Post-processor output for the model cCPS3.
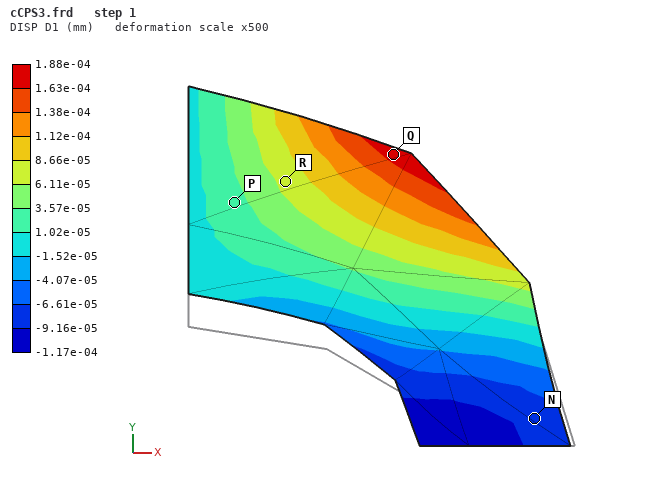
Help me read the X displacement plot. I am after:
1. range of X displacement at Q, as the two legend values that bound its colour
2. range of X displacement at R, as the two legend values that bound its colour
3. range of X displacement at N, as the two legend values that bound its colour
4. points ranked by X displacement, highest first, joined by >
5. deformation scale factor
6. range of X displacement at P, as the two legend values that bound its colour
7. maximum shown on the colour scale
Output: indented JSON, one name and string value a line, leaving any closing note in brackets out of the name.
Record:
{
  "range of X displacement at Q, as the two legend values that bound its colour": "1.63e-04 to 1.88e-04 mm",
  "range of X displacement at R, as the two legend values that bound its colour": "6.11e-05 to 8.66e-05 mm",
  "range of X displacement at N, as the two legend values that bound its colour": "-9.16e-05 to -6.61e-05 mm",
  "points ranked by X displacement, highest first, joined by >": "Q > R > P > N",
  "deformation scale factor": "500",
  "range of X displacement at P, as the two legend values that bound its colour": "1.02e-05 to 3.57e-05 mm",
  "maximum shown on the colour scale": "1.88e-04 mm"
}
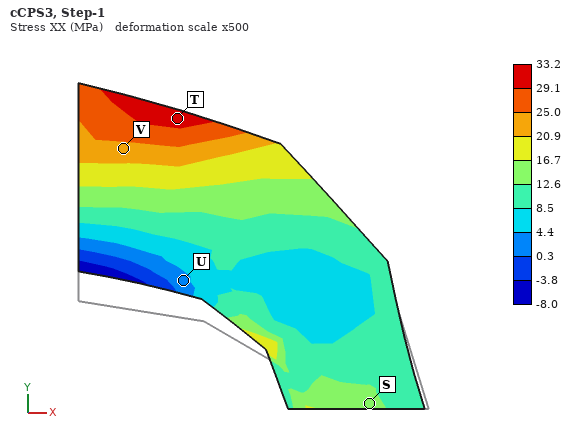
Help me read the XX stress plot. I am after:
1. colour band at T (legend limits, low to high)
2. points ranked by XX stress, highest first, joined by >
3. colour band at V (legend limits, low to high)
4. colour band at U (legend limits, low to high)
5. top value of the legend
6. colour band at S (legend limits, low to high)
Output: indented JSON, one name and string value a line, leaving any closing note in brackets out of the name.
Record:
{
  "colour band at T": "29.1 to 33.2 MPa",
  "points ranked by XX stress, highest first, joined by >": "T > V > S > U",
  "colour band at V": "20.9 to 25.0 MPa",
  "colour band at U": "0.3 to 4.4 MPa",
  "top value of the legend": "33.2 MPa",
  "colour band at S": "12.6 to 16.7 MPa"
}
